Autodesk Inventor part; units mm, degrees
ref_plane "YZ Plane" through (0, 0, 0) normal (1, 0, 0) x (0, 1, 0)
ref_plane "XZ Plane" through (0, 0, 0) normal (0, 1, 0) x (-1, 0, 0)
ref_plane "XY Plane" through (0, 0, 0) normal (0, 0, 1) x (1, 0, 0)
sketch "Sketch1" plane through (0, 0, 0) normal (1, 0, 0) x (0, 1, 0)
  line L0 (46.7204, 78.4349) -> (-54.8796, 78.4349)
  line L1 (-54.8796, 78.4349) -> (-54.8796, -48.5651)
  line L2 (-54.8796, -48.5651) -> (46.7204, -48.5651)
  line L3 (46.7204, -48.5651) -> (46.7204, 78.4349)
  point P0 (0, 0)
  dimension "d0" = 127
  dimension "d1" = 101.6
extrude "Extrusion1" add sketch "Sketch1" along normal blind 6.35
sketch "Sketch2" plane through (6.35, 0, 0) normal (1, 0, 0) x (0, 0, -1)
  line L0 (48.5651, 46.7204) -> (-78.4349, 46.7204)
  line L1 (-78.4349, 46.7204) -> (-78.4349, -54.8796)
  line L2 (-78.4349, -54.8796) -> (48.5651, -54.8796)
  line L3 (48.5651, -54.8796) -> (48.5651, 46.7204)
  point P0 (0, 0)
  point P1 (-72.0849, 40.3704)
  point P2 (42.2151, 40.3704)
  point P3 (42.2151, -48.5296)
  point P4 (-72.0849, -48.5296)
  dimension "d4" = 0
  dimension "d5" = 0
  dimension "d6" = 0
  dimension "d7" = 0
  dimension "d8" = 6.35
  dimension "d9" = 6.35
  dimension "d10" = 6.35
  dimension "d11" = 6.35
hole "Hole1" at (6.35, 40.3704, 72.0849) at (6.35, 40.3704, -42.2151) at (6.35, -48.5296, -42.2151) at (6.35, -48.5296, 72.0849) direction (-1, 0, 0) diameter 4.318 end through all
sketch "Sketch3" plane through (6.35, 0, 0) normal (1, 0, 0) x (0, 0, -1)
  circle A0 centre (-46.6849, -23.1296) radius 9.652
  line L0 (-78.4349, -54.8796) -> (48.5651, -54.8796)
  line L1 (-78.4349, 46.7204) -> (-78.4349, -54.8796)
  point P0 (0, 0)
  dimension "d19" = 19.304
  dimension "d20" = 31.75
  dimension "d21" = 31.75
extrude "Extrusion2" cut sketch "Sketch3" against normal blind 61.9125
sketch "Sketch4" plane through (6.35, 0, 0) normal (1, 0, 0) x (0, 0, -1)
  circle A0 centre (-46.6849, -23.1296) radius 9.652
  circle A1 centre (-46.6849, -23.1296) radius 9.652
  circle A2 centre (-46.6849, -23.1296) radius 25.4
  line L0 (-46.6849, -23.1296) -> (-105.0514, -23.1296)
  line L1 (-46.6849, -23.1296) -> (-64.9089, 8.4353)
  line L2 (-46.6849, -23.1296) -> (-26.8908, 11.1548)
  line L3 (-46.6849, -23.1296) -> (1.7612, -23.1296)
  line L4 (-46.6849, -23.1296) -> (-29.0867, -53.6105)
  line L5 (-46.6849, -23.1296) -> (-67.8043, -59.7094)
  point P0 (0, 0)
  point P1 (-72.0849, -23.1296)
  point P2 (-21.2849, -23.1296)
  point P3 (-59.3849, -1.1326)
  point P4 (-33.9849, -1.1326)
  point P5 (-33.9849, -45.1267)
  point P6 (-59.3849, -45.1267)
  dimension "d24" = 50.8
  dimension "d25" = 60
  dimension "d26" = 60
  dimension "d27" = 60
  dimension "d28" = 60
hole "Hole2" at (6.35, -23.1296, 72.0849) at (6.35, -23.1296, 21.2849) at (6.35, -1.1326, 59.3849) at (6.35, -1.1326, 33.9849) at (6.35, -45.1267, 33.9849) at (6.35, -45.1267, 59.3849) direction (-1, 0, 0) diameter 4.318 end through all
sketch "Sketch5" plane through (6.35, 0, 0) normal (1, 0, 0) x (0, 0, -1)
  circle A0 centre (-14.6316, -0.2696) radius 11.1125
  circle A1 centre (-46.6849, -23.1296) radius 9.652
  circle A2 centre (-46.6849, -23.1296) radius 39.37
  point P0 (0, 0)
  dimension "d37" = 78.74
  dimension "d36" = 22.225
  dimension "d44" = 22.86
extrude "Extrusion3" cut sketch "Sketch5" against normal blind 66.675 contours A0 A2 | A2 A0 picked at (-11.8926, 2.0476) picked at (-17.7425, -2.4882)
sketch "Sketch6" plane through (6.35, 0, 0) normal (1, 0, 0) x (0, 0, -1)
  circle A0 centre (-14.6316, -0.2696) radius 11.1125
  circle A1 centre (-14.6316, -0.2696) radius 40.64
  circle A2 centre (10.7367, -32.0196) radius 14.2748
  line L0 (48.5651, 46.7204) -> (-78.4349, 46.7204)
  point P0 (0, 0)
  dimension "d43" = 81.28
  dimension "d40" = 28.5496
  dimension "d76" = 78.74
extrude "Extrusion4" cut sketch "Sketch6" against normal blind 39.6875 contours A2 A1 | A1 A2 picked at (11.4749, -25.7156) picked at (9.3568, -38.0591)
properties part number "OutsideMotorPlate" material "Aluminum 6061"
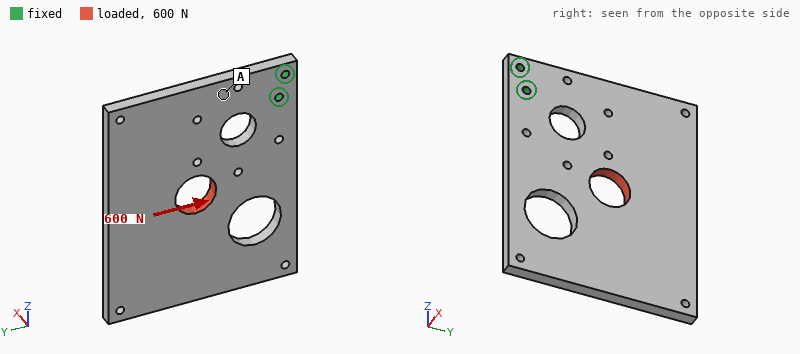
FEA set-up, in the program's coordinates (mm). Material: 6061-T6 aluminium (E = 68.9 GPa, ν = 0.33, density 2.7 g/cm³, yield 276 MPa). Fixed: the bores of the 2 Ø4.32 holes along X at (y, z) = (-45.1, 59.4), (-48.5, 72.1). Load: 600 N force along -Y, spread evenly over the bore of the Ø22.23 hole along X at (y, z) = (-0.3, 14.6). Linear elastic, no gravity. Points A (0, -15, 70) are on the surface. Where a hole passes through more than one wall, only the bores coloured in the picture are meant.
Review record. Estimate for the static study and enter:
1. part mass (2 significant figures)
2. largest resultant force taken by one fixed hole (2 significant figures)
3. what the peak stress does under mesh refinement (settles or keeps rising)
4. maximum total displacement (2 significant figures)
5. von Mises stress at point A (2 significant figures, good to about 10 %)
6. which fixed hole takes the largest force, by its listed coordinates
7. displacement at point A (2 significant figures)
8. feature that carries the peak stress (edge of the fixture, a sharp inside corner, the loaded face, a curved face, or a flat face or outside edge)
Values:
200 g
2.1 kN
keeps rising
0.12 mm
5.1 MPa
(-45.1, 59.4)
0.021 mm
edge of the fixture
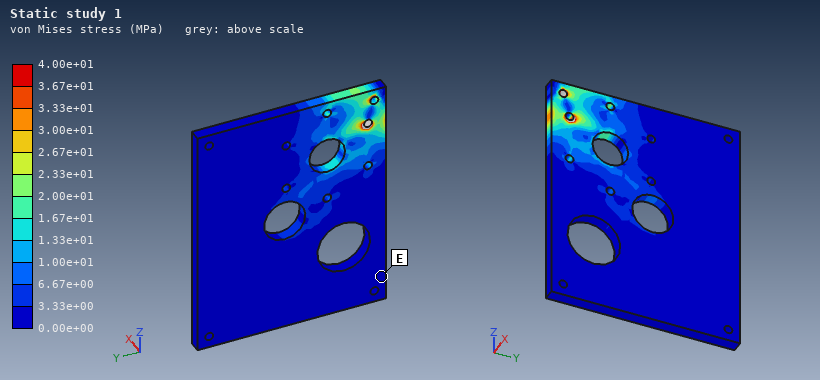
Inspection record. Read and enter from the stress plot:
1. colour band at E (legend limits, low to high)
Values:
0.00e+00 to 3.33e+00 MPa
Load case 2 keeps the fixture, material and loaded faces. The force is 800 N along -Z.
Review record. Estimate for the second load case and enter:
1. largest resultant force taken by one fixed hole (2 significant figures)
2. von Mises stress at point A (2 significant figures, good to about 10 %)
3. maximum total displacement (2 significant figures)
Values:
2.3 kN
7.7 MPa
0.14 mm
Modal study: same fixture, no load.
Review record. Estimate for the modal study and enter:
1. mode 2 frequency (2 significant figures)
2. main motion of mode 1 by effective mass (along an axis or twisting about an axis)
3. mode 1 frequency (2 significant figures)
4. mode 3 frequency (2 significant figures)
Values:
490 Hz
along X
240 Hz
850 Hz
